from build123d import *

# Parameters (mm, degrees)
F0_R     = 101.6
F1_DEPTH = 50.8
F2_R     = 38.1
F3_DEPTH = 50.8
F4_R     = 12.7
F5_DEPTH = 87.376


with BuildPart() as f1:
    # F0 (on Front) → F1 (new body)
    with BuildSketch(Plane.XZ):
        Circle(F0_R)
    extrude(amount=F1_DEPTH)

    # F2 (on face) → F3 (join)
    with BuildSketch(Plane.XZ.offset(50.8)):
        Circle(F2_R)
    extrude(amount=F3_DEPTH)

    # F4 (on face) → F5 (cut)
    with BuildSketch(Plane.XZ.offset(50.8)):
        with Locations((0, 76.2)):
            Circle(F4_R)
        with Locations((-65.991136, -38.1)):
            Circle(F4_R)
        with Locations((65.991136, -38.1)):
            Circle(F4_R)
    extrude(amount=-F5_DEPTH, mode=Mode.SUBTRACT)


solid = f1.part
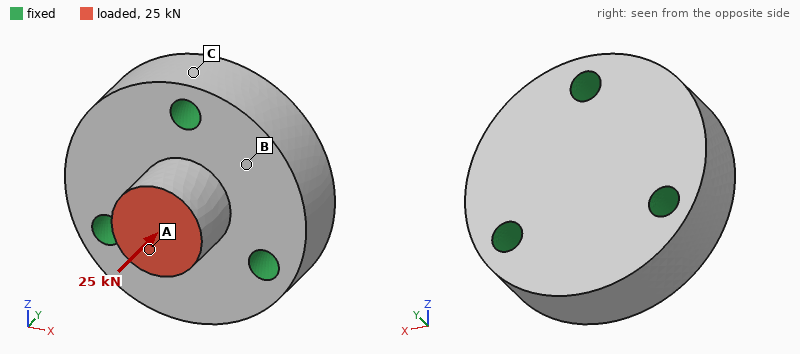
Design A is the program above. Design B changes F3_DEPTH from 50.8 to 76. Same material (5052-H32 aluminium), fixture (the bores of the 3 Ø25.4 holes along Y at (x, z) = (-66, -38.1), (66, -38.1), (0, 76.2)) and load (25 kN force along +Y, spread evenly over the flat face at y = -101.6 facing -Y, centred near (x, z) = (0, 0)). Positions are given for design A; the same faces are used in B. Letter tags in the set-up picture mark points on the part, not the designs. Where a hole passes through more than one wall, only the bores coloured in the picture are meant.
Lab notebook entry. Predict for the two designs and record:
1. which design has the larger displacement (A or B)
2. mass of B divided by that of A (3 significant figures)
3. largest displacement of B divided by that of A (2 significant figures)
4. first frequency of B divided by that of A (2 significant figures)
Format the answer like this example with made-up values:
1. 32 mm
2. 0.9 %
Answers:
1. B
2. 1.06
3. 1.2
4. 0.71
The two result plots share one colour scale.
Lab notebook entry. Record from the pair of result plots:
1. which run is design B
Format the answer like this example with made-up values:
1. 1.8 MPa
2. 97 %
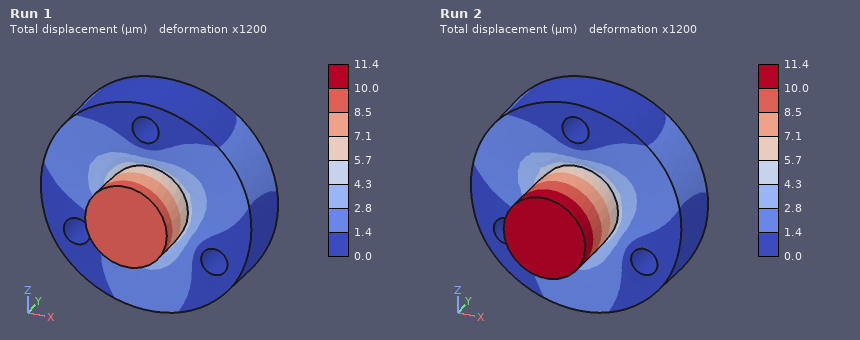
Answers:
1. Run 2
